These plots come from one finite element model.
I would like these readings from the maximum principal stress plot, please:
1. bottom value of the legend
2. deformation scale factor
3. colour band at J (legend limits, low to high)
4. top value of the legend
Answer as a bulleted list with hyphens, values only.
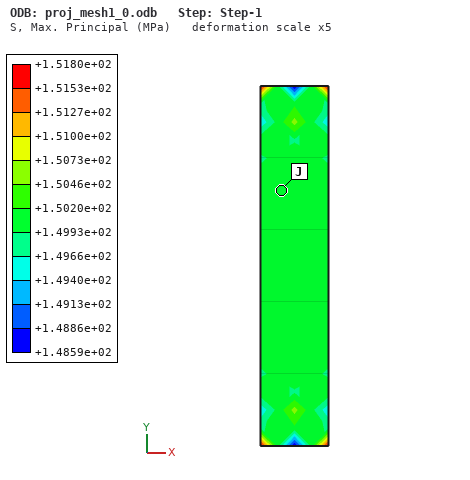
- +1.4859e+02 MPa
- 5
- +1.4993e+02 to +1.5020e+02 MPa
- +1.5180e+02 MPa
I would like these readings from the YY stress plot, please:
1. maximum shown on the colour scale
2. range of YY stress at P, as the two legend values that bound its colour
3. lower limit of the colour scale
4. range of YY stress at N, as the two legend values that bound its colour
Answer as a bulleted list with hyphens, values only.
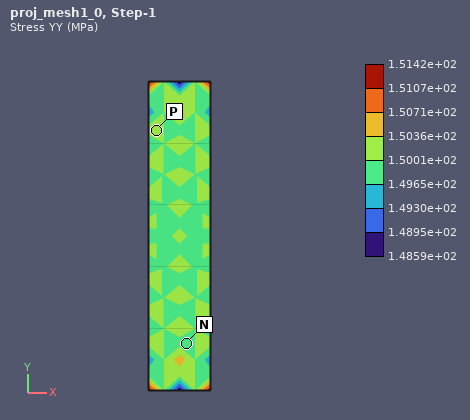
- 1.5142e+02 MPa
- 1.5001e+02 to 1.5036e+02 MPa
- 1.4859e+02 MPa
- 1.4965e+02 to 1.5001e+02 MPa
